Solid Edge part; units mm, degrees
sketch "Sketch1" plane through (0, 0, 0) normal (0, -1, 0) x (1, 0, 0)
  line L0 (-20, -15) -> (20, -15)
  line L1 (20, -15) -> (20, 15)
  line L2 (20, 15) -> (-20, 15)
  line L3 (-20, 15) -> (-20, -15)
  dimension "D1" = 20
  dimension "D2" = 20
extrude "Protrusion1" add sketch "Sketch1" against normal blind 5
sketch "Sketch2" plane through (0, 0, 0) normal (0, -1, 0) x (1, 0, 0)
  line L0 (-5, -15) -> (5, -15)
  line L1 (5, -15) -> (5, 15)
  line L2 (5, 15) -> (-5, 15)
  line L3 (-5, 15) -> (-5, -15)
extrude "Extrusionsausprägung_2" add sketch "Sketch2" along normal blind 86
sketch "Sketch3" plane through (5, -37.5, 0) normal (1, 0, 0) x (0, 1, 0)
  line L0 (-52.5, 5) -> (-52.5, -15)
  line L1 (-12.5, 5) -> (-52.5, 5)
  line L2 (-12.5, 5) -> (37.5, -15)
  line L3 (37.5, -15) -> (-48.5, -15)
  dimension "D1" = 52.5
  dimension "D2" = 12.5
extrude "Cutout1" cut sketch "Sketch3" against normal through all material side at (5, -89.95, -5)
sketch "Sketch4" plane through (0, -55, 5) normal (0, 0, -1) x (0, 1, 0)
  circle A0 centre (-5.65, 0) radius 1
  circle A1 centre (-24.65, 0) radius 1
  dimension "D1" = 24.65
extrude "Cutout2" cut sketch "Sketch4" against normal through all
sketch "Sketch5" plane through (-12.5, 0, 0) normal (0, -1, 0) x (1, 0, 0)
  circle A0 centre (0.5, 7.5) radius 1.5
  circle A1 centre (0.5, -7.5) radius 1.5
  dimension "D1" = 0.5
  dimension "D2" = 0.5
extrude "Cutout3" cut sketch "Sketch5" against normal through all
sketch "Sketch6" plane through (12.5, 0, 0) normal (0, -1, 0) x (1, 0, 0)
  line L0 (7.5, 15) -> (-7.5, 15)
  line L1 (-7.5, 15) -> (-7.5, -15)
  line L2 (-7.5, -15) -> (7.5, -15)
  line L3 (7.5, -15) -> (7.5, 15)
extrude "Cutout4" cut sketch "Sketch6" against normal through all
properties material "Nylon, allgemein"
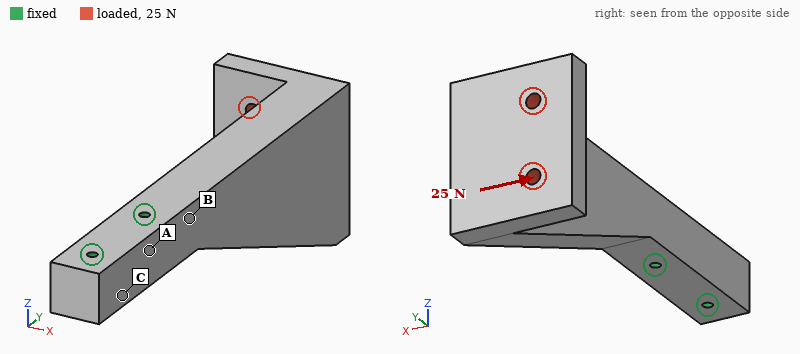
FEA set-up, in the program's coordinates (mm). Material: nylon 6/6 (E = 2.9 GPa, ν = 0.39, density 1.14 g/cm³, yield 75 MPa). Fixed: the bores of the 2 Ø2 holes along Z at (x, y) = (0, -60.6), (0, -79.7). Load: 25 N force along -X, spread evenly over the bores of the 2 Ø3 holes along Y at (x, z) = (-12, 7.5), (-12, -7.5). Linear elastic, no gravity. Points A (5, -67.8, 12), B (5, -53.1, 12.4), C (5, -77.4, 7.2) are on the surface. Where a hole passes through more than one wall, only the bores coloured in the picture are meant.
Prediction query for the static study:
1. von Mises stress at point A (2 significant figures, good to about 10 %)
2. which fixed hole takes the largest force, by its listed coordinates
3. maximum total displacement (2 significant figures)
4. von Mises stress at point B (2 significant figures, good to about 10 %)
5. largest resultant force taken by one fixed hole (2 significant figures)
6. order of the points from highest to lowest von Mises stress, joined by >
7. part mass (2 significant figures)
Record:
3.9 MPa
(0, -60.6)
1.2 mm
8.3 MPa
87 N
B > A > C
20 g
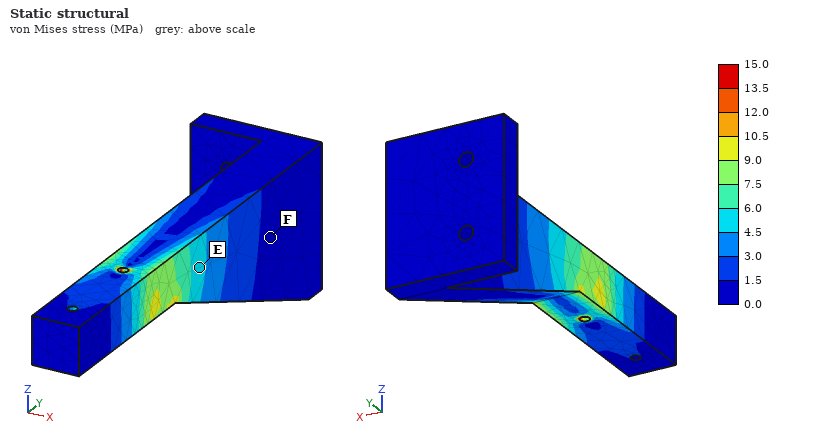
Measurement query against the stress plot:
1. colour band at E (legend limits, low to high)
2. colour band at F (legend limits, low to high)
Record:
4.5 to 6.0 MPa
0.0 to 1.5 MPa
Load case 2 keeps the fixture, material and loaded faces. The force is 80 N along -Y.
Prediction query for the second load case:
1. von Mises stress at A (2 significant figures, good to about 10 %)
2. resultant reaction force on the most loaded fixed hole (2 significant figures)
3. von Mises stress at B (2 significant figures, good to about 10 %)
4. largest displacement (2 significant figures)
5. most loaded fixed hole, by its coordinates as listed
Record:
2.5 MPa
82 N
7.1 MPa
1.1 mm
(0, -60.6)
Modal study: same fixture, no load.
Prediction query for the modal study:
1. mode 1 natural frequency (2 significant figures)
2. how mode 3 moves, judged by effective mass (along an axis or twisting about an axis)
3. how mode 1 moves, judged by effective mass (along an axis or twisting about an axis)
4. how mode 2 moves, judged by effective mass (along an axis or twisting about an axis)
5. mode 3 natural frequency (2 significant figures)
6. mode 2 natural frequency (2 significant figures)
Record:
270 Hz
twisting about Y
along X
along Z
1100 Hz
320 Hz
